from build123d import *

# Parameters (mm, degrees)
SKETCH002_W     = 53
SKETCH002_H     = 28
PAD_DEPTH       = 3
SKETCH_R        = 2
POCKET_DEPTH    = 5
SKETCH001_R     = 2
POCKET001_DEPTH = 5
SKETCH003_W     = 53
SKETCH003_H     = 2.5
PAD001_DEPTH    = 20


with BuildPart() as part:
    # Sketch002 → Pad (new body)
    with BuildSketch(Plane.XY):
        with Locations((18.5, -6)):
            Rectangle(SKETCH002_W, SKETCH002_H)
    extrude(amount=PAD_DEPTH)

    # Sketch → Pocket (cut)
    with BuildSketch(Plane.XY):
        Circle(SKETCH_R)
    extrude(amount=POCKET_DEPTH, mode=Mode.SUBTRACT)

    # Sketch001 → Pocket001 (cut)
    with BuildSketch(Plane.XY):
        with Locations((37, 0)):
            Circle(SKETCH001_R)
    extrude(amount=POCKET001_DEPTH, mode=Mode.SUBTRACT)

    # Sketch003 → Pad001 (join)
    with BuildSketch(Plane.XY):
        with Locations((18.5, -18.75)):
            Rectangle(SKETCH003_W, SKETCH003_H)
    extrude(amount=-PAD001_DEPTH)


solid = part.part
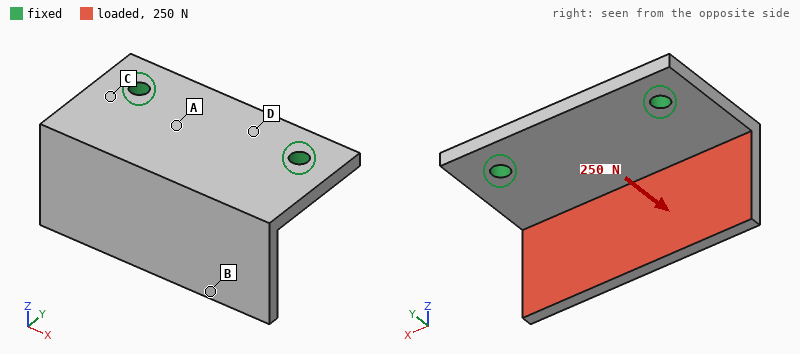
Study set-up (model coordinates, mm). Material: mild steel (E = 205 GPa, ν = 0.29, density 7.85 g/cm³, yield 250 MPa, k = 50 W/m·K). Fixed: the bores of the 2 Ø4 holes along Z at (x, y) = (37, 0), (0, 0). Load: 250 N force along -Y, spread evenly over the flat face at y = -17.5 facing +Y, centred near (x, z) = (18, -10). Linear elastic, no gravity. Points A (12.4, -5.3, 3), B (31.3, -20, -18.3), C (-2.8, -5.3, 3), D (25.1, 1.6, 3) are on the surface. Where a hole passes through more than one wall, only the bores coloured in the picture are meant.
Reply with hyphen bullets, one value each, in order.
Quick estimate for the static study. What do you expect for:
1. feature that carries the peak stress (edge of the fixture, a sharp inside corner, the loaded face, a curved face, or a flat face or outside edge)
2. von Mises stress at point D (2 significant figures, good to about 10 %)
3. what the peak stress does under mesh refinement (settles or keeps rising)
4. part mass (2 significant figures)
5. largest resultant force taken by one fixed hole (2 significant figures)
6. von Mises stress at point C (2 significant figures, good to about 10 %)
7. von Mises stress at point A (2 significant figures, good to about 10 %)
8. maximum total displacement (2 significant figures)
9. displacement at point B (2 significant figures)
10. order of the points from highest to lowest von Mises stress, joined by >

- edge of the fixture
- 12 MPa
- keeps rising
- 55 g
- 130 N
- 40 MPa
- 23 MPa
- 72 µm
- 67 µm
- C > A > D > B
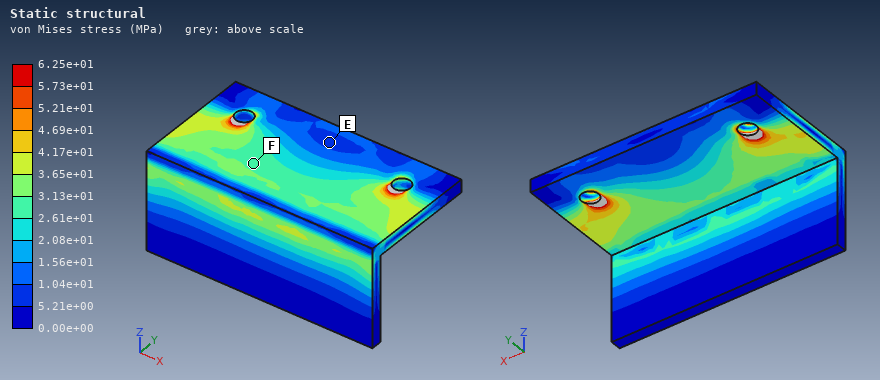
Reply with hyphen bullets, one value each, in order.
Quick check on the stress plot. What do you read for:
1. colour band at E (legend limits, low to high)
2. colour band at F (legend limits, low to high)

- 5.21e+00 to 1.04e+01 MPa
- 2.61e+01 to 3.13e+01 MPa
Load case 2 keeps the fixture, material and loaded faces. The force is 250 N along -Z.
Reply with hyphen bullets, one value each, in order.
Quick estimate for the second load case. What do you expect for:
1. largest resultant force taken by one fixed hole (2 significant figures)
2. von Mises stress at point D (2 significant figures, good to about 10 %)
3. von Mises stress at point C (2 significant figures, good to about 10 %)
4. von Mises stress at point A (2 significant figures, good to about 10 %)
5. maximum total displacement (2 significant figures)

- 130 N
- 16 MPa
- 48 MPa
- 22 MPa
- 43 µm
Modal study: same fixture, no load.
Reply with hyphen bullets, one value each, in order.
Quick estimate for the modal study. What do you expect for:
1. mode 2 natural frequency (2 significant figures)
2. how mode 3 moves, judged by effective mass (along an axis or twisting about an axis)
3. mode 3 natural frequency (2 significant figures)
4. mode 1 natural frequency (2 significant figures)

- 3600 Hz
- along Z
- 5100 Hz
- 2100 Hz
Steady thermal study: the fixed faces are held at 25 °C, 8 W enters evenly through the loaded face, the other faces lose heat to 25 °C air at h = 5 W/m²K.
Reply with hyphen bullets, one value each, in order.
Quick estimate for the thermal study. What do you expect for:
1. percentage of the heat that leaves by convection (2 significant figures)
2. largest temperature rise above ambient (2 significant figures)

- 4.7 %
- 34 K
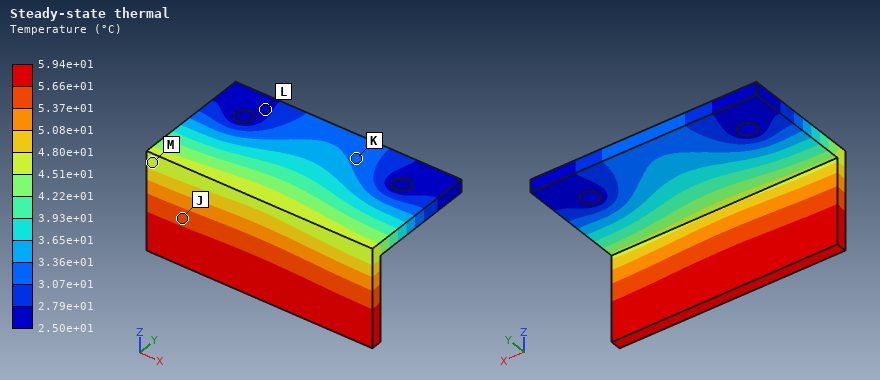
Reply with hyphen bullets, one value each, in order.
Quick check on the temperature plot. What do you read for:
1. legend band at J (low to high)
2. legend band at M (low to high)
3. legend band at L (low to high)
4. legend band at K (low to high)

- 5.37e+01 to 5.66e+01 °C
- 4.51e+01 to 4.80e+01 °C
- 2.50e+01 to 2.79e+01 °C
- 3.07e+01 to 3.36e+01 °C
